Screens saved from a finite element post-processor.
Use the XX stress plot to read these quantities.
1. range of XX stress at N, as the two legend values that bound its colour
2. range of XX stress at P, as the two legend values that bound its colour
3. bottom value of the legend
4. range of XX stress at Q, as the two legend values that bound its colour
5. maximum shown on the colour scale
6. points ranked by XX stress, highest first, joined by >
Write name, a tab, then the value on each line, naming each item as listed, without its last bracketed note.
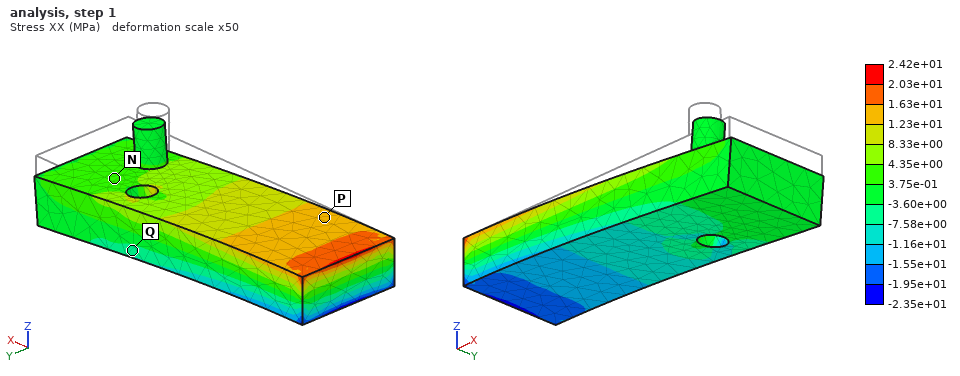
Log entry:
range of XX stress at N, as the two legend values that bound its colour	3.75e-01 to 4.35e+00 MPa
range of XX stress at P, as the two legend values that bound its colour	1.23e+01 to 1.63e+01 MPa
bottom value of the legend	-2.35e+01 MPa
range of XX stress at Q, as the two legend values that bound its colour	-7.58e+00 to -3.60e+00 MPa
maximum shown on the colour scale	2.42e+01 MPa
points ranked by XX stress, highest first, joined by >	P > N > Q
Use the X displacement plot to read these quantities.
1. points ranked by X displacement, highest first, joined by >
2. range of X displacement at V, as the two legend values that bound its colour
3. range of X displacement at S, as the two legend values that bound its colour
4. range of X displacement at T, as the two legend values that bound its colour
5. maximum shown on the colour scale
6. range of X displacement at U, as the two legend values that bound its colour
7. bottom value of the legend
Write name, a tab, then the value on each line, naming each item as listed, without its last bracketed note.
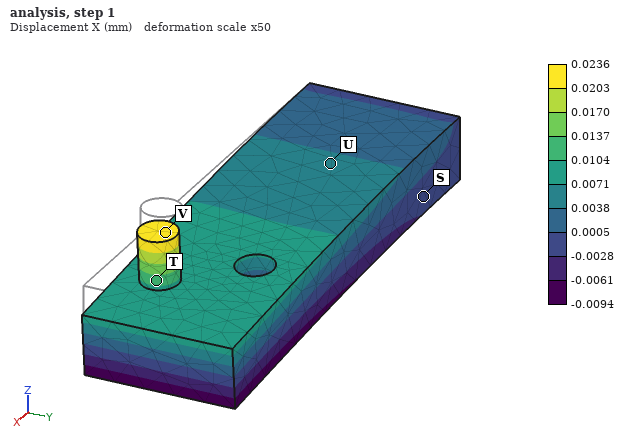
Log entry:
points ranked by X displacement, highest first, joined by >	V > T > U > S
range of X displacement at V, as the two legend values that bound its colour	0.0203 to 0.0236 mm
range of X displacement at S, as the two legend values that bound its colour	-0.0028 to 0.0005 mm
range of X displacement at T, as the two legend values that bound its colour	0.0104 to 0.0137 mm
maximum shown on the colour scale	0.0236 mm
range of X displacement at U, as the two legend values that bound its colour	0.0038 to 0.0071 mm
bottom value of the legend	-0.0094 mm
